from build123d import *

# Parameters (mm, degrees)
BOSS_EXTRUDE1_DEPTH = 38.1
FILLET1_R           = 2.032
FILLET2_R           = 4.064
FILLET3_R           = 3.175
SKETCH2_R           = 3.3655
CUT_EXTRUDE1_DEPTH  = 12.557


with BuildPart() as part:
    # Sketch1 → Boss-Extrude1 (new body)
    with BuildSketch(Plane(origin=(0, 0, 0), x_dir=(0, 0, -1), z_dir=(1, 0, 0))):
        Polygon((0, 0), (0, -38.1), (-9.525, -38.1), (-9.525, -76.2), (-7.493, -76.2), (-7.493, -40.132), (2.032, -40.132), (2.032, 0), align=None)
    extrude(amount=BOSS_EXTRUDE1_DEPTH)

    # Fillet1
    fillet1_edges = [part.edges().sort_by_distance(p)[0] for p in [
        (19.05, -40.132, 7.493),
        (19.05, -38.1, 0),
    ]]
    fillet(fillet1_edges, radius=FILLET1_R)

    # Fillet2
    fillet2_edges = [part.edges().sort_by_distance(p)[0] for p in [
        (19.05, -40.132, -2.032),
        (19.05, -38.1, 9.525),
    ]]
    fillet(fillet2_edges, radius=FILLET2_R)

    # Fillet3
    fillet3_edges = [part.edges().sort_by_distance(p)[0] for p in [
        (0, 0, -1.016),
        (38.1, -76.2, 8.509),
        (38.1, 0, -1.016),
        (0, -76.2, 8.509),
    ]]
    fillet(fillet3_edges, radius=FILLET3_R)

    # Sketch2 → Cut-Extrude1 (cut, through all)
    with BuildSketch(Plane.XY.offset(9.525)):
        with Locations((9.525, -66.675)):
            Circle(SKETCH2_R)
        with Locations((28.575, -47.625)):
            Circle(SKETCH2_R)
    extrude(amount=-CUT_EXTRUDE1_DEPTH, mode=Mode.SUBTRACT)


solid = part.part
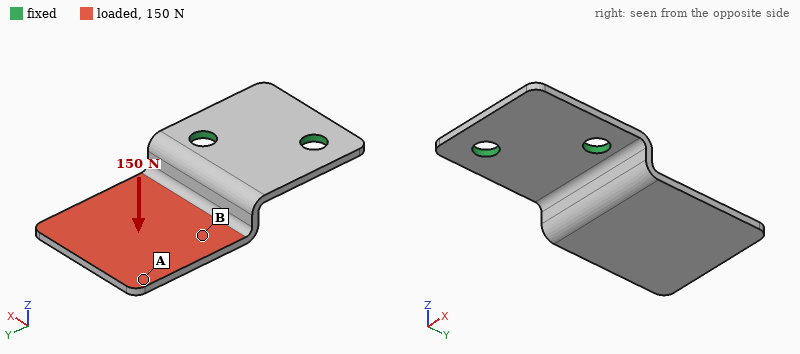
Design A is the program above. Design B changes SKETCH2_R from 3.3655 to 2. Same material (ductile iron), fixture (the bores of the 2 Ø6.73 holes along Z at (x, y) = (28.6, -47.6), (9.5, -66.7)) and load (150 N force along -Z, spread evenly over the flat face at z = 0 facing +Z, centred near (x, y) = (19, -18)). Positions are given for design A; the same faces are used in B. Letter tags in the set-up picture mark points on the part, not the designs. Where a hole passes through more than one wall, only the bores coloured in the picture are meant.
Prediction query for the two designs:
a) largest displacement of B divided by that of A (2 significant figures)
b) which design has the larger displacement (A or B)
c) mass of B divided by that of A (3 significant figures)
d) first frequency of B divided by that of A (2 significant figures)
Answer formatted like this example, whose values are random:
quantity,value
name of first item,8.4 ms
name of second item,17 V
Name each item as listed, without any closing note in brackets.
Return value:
quantity,value
largest displacement of B divided by that of A,1.1
which design has the larger displacement,B
mass of B divided by that of A,1.01
first frequency of B divided by that of A,0.93
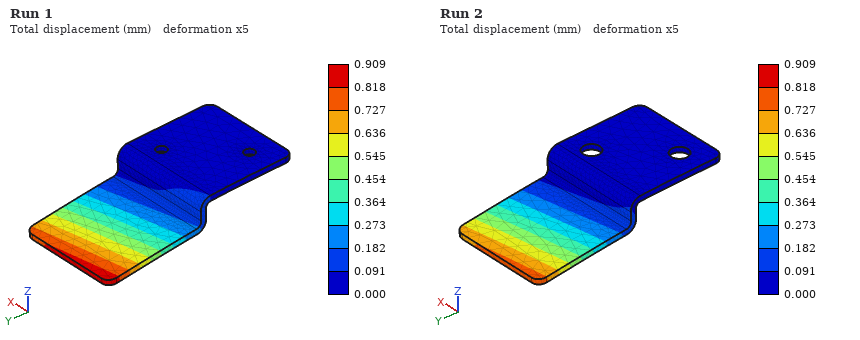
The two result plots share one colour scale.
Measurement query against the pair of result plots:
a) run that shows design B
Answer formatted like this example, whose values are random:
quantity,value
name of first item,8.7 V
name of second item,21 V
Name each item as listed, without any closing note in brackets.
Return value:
quantity,value
run that shows design B,Run 1
